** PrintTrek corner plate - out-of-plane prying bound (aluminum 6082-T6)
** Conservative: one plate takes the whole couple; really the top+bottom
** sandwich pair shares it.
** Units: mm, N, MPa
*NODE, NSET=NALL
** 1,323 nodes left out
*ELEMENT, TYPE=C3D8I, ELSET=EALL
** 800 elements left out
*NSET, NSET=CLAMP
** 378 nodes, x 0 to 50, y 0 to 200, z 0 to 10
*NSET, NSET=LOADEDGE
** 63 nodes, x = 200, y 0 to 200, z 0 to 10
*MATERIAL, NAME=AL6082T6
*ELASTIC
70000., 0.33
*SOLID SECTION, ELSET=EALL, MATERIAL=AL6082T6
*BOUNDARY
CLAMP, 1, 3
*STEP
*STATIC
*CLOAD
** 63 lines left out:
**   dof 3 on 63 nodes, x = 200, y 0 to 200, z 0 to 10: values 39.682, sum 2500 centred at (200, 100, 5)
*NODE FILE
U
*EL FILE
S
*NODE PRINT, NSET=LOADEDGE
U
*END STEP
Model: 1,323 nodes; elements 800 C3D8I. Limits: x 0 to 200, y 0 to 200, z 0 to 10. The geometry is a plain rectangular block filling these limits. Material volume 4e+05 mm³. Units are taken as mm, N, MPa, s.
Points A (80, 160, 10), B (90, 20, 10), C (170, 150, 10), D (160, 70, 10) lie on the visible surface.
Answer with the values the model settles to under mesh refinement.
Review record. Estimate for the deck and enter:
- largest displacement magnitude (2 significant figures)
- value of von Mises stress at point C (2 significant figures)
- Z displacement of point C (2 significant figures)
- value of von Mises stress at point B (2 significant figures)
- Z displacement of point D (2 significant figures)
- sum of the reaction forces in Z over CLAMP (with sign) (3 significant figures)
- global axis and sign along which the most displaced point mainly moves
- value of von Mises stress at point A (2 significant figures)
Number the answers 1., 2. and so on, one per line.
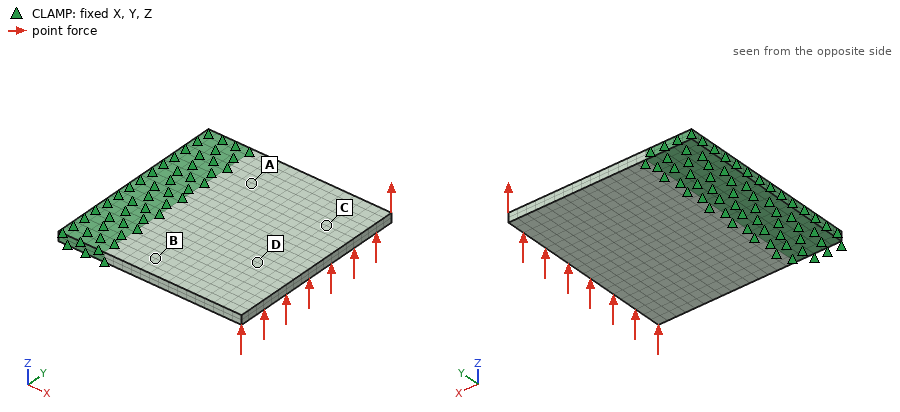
1. 2.2 mm
2. 22 MPa
3. 1.6 mm
4. 77 MPa
5. 1.4 mm
6. -2500 N
7. +Z
8. 80 MPa
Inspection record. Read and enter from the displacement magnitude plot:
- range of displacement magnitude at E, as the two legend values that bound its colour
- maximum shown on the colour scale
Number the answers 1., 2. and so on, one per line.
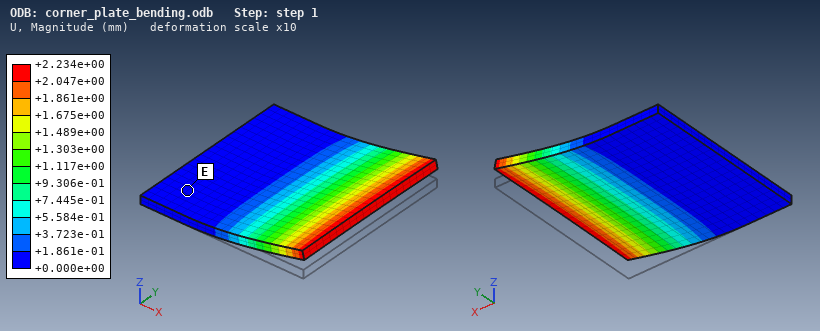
1. +0.000e+00 to +1.861e-01 mm
2. +2.234e+00 mm
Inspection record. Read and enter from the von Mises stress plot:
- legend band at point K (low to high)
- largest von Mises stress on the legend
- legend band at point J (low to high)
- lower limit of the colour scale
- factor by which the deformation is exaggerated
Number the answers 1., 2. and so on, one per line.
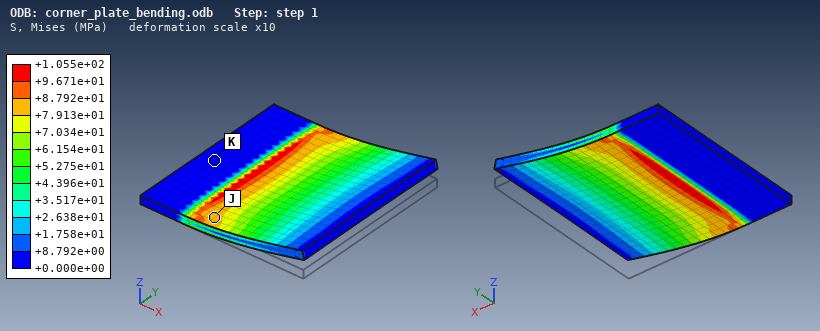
1. +0.000e+00 to +8.792e+00 MPa
2. +1.055e+02 MPa
3. +7.913e+01 to +8.792e+01 MPa
4. +0.000e+00 MPa
5. 10
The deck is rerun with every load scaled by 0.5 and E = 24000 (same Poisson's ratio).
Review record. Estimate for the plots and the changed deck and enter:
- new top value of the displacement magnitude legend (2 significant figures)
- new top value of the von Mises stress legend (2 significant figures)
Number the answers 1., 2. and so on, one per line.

1. 3.3 mm
2. 53 MPa
